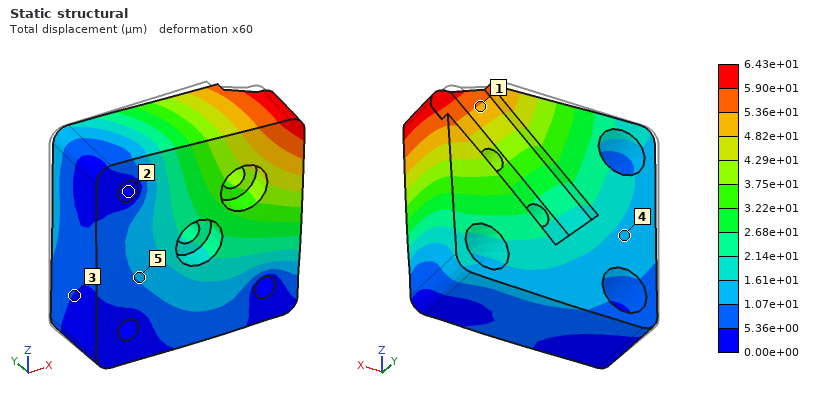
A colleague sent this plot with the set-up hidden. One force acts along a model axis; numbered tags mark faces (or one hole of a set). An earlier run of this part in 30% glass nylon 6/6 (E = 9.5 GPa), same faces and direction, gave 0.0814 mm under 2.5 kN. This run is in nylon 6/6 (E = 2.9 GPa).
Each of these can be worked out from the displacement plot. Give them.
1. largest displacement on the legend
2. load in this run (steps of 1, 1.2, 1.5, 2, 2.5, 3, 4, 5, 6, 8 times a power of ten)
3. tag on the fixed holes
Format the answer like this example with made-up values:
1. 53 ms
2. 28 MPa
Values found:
1. 6.43e+01 µm
2. 600 N
3. 2
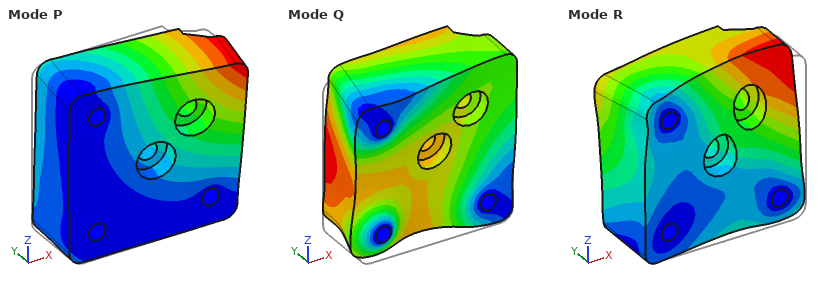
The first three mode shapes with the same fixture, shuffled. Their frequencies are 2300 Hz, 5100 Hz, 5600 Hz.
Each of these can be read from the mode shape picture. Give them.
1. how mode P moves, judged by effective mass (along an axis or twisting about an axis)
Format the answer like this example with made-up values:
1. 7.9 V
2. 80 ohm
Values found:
1. along Y
